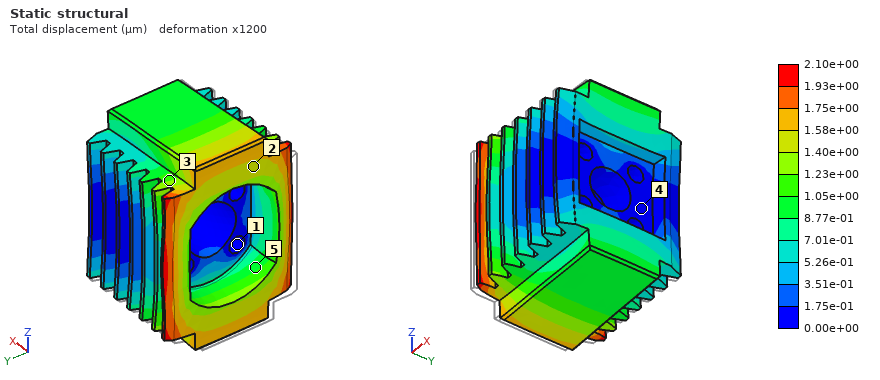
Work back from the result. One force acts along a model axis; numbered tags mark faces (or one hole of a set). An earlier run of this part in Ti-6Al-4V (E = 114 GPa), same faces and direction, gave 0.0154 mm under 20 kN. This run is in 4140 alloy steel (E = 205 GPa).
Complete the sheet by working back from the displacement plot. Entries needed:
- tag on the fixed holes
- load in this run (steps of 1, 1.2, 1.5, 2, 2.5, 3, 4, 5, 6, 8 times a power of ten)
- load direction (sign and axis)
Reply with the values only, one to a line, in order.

1
5 kN
+X
